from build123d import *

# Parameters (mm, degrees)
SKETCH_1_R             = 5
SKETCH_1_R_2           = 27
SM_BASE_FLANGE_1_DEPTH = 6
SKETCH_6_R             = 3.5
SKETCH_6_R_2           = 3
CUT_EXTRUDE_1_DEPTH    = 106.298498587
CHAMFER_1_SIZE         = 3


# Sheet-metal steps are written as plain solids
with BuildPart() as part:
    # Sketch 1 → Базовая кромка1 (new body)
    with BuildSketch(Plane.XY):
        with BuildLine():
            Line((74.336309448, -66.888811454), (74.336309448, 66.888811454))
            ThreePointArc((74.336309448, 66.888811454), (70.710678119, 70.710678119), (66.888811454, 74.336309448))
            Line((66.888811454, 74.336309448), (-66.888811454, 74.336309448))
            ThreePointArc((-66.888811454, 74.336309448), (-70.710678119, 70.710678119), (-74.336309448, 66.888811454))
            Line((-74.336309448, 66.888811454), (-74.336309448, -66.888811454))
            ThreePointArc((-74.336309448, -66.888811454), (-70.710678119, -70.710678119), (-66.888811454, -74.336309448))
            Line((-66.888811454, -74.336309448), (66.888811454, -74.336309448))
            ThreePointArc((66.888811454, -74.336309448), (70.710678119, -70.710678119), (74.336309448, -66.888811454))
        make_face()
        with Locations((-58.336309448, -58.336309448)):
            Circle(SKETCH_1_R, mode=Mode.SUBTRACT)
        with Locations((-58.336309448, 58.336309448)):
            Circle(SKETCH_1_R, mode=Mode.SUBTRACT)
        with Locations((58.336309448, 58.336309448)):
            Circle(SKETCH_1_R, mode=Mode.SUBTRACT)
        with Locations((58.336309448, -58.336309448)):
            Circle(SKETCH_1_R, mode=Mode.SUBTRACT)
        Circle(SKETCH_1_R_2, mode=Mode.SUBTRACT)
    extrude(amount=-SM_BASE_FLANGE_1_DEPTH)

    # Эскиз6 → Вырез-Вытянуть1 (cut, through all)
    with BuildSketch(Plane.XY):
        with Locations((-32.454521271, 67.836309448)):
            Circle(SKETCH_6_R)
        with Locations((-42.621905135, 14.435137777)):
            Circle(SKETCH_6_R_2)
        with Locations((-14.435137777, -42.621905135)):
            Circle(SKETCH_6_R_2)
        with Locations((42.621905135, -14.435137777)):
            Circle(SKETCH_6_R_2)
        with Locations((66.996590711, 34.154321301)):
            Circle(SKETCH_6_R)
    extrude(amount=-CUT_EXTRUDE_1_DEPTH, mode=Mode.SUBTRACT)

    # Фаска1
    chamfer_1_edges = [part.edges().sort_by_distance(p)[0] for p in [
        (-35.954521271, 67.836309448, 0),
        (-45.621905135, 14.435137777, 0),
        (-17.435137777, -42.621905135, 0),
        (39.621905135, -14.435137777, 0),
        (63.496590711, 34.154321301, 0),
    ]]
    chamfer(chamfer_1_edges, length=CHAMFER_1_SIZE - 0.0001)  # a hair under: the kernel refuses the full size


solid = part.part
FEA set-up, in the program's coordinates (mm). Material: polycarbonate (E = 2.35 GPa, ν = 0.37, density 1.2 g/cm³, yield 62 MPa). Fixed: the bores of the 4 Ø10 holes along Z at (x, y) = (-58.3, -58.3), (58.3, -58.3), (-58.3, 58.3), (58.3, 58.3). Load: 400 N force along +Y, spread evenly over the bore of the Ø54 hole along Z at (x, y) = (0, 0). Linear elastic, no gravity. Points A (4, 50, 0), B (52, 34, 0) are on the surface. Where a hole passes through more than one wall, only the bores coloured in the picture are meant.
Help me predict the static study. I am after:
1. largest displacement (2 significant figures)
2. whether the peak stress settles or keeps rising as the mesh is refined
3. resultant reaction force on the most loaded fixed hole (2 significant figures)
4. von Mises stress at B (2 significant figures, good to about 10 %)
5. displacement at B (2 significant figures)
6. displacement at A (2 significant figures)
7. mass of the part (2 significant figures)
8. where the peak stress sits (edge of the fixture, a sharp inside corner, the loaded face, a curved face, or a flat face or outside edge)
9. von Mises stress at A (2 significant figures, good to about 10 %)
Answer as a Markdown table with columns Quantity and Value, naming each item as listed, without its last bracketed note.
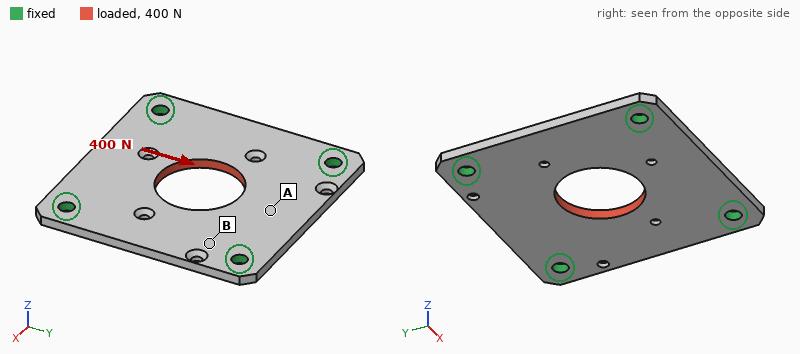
| Quantity | Value |
|---|---|
| largest displacement | 20 µm |
| whether the peak stress settles or keeps rising as the mesh is refined | keeps rising |
| resultant reaction force on the most loaded fixed hole | 110 N |
| von Mises stress at B | 0.44 MPa |
| displacement at B | 5.3 µm |
| displacement at A | 17 µm |
| mass of the part | 140 g |
| where the peak stress sits | edge of the fixture |
| von Mises stress at A | 0.18 MPa |
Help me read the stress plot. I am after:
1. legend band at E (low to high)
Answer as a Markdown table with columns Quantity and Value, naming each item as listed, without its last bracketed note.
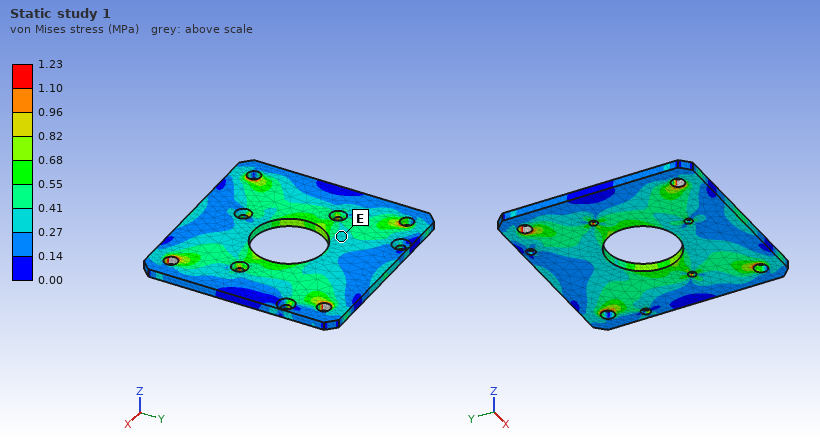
| Quantity | Value |
|---|---|
| legend band at E | 0.27 to 0.41 MPa |
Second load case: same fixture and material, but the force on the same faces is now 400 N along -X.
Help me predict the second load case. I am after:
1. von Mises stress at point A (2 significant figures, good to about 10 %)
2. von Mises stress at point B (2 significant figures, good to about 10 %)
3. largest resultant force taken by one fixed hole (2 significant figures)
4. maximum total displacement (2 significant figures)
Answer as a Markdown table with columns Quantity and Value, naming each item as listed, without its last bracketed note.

| Quantity | Value |
|---|---|
| von Mises stress at point A | 0.34 MPa |
| von Mises stress at point B | 0.45 MPa |
| largest resultant force taken by one fixed hole | 110 N |
| maximum total displacement | 20 µm |
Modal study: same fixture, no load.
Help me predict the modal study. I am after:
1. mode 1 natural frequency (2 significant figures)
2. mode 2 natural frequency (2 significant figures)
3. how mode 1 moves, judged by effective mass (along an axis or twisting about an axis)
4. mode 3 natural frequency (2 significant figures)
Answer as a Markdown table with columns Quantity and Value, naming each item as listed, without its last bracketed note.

| Quantity | Value |
|---|---|
| mode 1 natural frequency | 500 Hz |
| mode 2 natural frequency | 710 Hz |
| how mode 1 moves, judged by effective mass | along Z |
| mode 3 natural frequency | 710 Hz |
